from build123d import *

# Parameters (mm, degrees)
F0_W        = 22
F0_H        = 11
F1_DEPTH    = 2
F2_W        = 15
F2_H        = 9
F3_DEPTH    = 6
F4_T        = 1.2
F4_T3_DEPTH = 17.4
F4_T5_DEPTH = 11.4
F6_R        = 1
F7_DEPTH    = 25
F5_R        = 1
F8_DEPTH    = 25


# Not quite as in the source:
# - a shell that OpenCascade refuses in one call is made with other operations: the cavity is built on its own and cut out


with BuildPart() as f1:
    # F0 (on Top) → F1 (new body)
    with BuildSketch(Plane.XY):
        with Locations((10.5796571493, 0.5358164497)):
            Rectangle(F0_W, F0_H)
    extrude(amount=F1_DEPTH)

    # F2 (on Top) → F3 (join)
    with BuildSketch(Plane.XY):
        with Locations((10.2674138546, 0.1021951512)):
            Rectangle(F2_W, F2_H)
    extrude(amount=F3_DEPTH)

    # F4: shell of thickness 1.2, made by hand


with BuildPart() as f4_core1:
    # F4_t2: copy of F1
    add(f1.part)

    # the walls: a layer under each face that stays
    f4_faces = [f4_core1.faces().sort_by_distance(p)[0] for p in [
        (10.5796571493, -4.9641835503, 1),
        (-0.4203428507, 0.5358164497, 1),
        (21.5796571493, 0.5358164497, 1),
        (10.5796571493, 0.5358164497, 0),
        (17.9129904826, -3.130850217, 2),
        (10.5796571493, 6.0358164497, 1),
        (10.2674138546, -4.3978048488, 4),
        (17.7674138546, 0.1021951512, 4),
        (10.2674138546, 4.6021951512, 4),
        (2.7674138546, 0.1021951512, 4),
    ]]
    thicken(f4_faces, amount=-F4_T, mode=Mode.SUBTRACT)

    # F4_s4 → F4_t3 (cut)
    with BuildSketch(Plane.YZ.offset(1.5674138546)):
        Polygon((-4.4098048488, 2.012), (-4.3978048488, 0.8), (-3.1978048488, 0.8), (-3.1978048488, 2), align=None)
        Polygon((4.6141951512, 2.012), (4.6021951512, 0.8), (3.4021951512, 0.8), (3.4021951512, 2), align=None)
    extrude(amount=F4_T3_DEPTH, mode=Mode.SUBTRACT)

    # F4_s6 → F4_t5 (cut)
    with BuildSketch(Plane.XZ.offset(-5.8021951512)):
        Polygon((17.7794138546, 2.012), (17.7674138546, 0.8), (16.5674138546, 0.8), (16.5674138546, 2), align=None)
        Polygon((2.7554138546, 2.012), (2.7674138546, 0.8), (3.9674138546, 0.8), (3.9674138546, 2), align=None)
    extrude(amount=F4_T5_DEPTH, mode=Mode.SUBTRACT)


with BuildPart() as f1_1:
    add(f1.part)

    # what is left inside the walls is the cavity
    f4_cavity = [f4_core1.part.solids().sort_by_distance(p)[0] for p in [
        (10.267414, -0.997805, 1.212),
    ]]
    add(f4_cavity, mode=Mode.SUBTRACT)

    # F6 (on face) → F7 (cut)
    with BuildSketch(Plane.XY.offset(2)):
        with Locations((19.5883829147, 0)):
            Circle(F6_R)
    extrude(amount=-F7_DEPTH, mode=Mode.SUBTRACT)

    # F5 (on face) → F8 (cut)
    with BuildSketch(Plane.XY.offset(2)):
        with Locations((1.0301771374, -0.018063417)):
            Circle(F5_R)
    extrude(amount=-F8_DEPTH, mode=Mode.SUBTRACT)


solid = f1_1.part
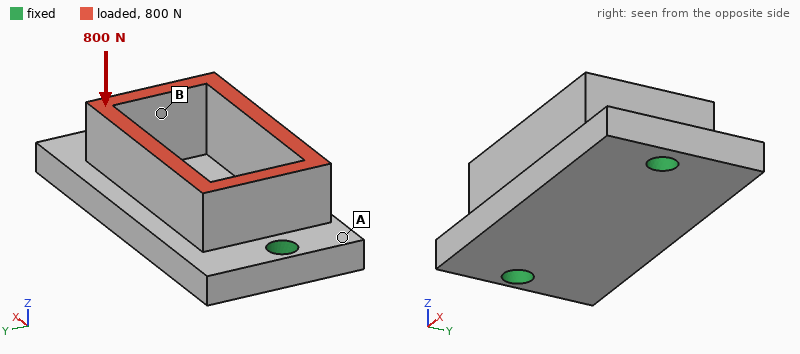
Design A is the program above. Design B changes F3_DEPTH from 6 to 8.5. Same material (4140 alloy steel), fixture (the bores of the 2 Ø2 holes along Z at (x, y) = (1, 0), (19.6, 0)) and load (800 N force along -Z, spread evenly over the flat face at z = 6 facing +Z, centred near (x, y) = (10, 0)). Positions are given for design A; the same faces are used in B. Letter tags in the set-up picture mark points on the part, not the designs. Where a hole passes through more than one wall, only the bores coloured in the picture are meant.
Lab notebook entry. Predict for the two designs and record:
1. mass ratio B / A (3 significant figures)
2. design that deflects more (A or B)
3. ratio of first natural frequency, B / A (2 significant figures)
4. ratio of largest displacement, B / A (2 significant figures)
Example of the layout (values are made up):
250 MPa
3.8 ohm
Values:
1.21
A
0.76
0.78
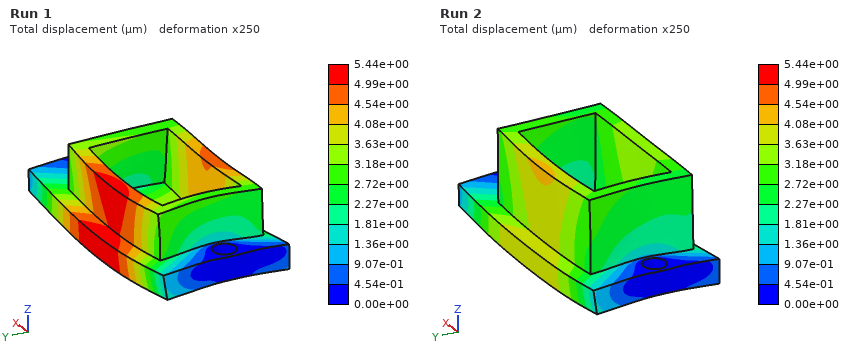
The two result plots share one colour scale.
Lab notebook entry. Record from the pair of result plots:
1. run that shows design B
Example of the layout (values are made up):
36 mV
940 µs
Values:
Run 2
